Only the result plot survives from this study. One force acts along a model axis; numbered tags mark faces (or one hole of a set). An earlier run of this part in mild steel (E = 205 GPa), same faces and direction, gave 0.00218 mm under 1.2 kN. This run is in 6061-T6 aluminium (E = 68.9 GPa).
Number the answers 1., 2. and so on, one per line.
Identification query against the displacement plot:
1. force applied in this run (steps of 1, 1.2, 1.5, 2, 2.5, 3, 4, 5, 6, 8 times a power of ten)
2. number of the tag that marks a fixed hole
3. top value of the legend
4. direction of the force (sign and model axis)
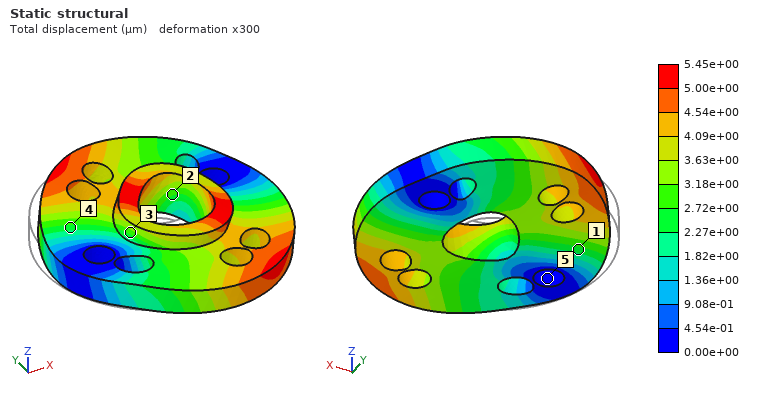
1. 1 kN
2. 5
3. 5.45e+00 µm
4. +X
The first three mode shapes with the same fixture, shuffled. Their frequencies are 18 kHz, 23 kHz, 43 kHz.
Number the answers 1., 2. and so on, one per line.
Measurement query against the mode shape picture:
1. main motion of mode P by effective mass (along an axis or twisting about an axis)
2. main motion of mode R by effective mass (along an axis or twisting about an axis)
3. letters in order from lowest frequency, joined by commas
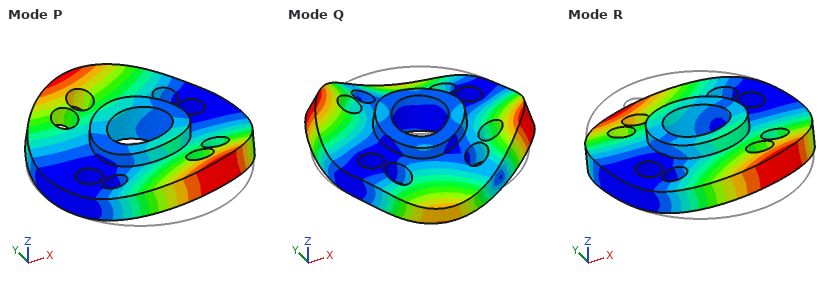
1. along Z
2. twisting about X
3. R, P, Q
